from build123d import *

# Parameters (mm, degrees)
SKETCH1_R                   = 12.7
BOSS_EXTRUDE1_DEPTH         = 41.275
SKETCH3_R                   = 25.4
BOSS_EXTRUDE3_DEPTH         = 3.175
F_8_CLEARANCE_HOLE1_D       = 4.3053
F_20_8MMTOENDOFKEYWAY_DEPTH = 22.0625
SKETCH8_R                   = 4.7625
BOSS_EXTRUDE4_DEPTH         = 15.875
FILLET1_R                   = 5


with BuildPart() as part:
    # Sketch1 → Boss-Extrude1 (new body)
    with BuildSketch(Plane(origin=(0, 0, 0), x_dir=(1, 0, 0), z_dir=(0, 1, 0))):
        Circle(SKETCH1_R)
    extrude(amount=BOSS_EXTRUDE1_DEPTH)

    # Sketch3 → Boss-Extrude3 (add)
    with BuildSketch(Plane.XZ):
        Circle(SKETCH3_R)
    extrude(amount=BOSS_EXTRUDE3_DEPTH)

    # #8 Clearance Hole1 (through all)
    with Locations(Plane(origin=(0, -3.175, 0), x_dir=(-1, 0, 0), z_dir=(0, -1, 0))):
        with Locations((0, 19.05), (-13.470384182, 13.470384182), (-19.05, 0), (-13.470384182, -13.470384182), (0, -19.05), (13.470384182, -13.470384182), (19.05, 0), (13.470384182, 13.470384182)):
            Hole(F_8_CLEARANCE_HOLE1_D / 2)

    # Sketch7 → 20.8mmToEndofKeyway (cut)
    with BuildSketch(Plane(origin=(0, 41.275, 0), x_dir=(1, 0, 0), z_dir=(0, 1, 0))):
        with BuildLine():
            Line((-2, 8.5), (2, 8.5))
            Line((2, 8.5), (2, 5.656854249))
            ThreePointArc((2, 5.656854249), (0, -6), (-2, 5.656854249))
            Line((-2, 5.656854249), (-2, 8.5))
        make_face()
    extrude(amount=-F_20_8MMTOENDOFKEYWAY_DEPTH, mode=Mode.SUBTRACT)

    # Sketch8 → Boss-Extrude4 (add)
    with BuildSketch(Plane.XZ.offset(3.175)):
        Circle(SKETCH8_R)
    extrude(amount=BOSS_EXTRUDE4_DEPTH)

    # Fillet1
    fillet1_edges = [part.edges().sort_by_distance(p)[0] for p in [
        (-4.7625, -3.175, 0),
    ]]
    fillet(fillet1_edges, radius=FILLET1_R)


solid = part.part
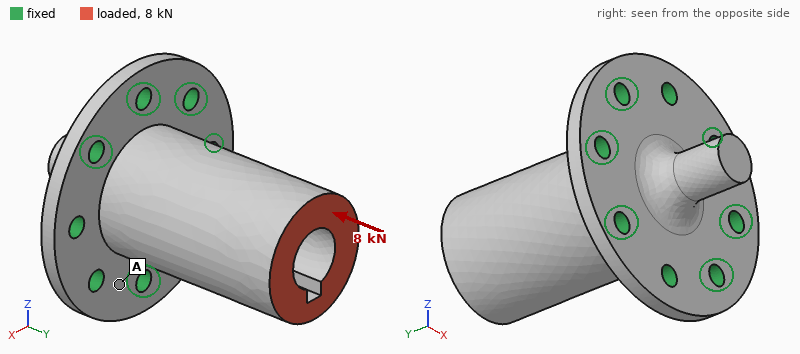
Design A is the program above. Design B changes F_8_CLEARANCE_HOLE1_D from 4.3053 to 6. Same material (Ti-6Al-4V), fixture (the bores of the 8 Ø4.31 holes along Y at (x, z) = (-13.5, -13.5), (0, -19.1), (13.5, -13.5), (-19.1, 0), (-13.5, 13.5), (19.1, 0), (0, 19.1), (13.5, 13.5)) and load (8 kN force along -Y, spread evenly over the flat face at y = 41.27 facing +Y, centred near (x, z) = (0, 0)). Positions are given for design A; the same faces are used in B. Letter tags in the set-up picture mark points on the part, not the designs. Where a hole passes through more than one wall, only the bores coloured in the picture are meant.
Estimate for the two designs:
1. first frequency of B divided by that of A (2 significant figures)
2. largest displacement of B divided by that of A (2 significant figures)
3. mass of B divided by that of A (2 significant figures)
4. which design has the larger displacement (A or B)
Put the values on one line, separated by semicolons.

1.1; 0.81; 0.99; A
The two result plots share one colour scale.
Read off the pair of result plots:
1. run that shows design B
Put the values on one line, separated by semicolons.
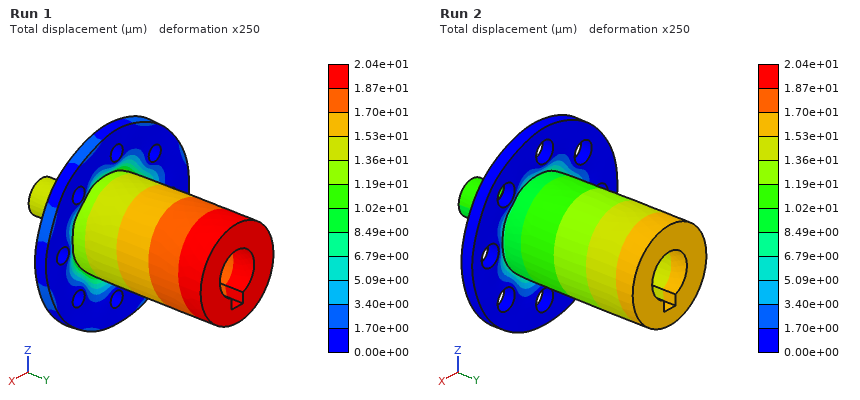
Run 2
